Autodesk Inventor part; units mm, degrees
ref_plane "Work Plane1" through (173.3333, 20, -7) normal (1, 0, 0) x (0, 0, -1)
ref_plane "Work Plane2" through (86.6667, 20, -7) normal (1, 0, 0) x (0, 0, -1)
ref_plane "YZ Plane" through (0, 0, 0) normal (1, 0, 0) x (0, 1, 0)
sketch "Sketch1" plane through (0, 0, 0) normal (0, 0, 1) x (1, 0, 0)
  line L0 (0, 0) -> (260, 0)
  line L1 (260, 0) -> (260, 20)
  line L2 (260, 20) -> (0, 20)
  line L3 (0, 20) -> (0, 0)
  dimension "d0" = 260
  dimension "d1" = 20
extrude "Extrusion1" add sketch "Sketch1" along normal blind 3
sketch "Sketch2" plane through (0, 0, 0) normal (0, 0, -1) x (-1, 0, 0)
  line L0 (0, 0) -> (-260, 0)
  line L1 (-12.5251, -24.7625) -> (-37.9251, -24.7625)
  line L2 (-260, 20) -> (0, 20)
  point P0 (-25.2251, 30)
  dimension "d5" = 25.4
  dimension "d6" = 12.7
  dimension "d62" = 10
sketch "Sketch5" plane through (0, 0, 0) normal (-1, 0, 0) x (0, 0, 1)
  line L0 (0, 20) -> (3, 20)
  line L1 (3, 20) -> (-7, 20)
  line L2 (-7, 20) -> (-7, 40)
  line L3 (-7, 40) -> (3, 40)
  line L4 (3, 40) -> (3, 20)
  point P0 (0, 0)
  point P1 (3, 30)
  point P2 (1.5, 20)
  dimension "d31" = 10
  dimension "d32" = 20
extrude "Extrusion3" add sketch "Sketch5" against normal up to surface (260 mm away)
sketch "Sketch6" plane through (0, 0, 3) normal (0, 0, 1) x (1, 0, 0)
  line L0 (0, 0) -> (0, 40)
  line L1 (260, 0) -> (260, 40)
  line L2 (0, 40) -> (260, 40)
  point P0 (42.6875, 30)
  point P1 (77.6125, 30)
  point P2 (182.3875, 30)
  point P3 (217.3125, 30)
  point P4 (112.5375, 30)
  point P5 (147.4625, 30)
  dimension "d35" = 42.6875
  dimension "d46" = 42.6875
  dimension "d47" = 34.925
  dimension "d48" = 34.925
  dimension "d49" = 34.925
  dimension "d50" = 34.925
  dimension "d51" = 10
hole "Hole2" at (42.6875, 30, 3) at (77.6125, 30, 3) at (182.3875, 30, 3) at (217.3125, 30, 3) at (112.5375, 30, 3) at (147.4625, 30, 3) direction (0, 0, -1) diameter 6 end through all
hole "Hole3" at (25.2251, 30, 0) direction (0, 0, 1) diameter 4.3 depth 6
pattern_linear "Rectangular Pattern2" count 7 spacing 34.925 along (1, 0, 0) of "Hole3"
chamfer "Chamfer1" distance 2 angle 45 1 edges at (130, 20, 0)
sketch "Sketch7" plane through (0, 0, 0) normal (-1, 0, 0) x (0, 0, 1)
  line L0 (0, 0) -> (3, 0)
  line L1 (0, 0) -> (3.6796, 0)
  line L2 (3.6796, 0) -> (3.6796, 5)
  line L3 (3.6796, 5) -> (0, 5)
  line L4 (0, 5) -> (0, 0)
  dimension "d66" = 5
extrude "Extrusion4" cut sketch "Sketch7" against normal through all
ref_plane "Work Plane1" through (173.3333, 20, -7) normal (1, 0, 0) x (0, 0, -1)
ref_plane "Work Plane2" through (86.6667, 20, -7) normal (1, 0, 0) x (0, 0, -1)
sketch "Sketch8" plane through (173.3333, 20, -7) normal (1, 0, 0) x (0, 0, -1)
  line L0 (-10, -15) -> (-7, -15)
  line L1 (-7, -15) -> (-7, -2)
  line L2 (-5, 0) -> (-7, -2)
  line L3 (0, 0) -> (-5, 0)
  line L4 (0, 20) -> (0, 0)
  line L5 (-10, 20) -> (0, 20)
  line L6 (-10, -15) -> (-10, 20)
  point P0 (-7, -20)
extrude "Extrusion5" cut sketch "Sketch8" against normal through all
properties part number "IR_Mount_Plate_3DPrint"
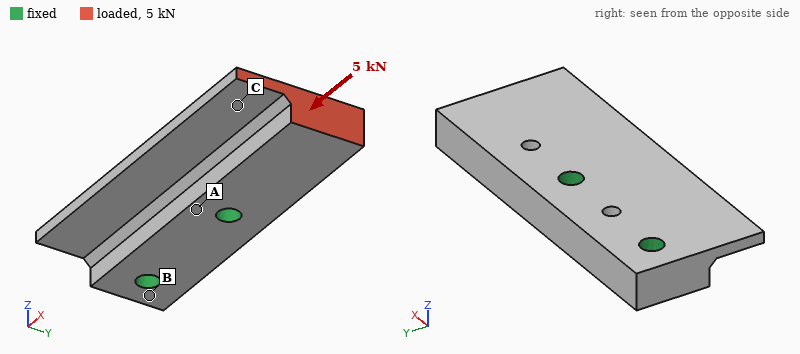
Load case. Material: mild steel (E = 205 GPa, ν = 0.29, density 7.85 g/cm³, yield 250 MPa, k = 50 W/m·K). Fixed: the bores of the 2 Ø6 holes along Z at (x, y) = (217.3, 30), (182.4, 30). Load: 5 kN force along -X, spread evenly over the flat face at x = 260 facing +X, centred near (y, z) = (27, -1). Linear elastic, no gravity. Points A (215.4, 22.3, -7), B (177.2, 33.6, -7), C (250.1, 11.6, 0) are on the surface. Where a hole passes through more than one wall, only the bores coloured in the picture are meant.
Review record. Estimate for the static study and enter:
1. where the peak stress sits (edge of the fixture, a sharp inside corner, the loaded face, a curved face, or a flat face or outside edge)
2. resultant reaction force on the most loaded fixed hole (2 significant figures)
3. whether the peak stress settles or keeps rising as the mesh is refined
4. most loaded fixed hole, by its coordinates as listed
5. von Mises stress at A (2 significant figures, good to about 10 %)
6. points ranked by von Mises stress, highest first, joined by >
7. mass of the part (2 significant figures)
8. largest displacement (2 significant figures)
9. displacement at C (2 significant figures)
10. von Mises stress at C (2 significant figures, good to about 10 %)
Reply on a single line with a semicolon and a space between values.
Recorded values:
edge of the fixture; 4.4 kN; keeps rising; (217.3, 30); 11 MPa; C > A > B; 160 g; 7.3 µm; 5.5 µm; 20 MPa
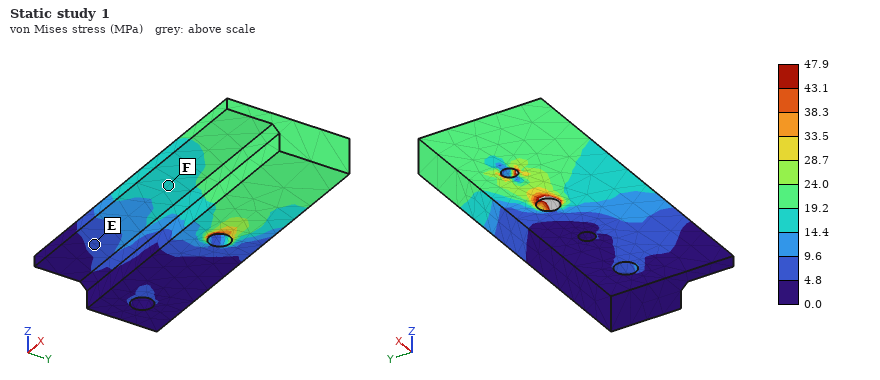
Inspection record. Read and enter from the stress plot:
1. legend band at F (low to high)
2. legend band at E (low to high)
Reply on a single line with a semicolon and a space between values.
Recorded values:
14.4 to 19.2 MPa; 4.8 to 9.6 MPa
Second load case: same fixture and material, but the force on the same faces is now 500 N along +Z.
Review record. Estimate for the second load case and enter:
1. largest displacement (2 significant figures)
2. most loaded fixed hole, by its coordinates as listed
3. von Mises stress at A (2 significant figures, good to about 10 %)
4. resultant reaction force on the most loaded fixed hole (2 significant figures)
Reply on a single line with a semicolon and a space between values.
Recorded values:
45 µm; (217.3, 30); 23 MPa; 620 N
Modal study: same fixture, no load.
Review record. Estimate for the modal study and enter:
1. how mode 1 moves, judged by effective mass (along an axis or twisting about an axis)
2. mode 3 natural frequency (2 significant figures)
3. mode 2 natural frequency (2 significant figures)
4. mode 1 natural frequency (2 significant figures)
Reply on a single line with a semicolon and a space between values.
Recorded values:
along Z; 7900 Hz; 7700 Hz; 4100 Hz
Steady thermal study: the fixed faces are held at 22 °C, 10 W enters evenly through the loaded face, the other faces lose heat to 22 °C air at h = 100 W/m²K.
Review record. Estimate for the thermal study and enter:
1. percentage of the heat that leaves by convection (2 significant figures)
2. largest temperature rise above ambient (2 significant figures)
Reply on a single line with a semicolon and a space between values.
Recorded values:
45 %; 25 K
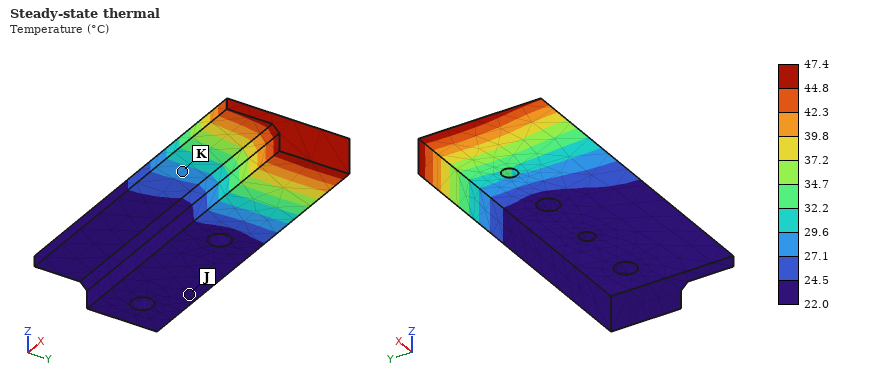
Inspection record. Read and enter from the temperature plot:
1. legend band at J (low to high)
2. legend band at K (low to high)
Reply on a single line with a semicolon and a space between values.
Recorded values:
22.0 to 24.5 °C; 27.1 to 29.6 °C
